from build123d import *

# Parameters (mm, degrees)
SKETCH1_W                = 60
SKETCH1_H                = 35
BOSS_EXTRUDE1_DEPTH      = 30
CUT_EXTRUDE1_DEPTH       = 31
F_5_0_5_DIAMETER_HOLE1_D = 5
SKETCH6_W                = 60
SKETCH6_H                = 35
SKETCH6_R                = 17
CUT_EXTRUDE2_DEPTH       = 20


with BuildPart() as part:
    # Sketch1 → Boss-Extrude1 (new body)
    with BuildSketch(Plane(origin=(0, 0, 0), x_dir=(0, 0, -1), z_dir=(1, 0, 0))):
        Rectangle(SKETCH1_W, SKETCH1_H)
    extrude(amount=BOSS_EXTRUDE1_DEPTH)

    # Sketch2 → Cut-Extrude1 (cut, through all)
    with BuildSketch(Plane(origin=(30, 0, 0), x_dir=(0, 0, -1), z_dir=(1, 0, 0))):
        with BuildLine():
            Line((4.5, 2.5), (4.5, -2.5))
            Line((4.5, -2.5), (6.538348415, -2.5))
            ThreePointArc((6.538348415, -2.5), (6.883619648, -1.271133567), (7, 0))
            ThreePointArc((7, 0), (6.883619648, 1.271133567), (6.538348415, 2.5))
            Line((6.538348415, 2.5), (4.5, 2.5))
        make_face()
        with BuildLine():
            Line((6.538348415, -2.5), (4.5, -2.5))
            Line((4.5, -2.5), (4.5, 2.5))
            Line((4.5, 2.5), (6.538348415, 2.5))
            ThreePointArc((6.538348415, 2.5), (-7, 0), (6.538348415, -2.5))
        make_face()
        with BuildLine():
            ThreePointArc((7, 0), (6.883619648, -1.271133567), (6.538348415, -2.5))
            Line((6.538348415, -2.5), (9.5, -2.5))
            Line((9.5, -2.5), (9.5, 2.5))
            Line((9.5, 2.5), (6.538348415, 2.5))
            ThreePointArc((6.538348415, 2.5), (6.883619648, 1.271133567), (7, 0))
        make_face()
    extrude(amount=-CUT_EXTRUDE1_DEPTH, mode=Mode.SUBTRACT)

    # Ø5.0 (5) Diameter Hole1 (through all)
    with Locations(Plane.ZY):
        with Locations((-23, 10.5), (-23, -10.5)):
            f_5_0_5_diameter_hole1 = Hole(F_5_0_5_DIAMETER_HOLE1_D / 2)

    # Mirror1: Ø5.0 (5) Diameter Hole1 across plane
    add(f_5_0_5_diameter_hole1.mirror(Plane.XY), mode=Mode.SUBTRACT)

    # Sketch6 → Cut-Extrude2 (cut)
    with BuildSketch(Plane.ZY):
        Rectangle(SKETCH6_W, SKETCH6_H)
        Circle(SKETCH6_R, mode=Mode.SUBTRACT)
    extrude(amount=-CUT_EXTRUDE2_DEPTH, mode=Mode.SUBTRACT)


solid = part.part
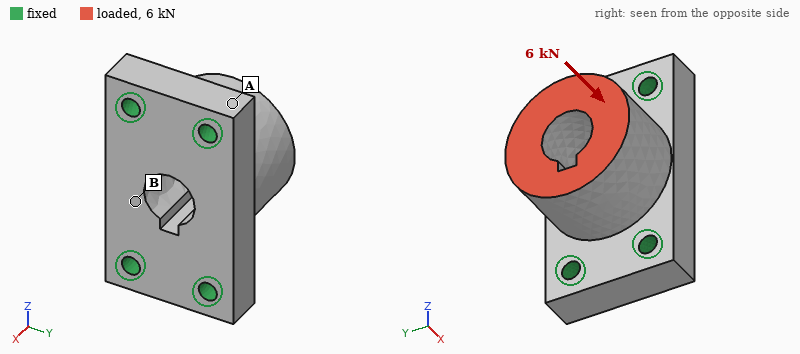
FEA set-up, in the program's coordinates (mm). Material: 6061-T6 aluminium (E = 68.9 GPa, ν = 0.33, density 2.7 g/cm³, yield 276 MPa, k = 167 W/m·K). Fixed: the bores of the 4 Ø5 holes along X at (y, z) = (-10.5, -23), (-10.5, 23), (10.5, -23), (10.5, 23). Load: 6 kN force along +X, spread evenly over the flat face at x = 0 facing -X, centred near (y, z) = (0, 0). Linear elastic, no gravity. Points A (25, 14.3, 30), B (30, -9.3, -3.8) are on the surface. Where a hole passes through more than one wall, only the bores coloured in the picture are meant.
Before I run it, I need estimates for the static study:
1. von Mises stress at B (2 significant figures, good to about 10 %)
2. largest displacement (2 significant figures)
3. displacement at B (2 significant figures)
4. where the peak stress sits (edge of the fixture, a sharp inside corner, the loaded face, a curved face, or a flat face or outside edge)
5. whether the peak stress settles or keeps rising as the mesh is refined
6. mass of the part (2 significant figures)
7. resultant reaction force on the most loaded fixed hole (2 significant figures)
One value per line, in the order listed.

13 MPa
11 µm
8.5 µm
edge of the fixture
keeps rising
90 g
1.6 kN
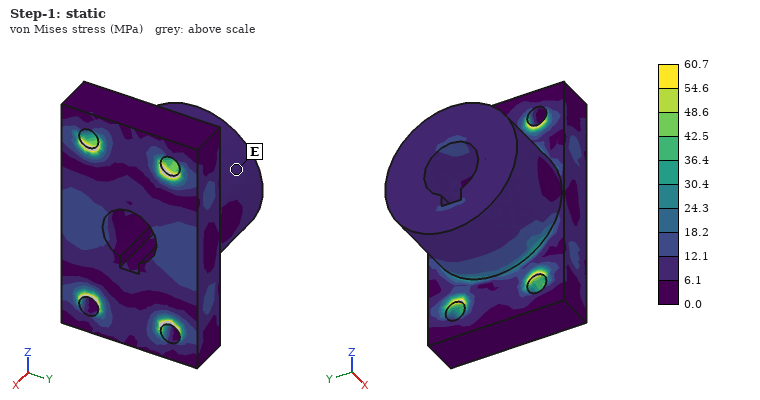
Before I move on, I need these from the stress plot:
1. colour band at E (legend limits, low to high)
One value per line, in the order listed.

6.1 to 12.1 MPa
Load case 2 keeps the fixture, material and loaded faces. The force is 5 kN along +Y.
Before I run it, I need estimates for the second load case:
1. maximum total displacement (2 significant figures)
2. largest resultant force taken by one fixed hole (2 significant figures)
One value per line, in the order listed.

56 µm
3.1 kN
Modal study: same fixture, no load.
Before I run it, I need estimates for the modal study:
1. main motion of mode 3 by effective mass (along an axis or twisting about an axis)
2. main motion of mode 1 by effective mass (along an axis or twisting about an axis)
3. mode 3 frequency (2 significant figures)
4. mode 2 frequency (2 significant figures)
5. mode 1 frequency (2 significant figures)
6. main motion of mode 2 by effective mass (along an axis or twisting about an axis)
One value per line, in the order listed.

along Z
along Y
18 kHz
17 kHz
11 kHz
along X
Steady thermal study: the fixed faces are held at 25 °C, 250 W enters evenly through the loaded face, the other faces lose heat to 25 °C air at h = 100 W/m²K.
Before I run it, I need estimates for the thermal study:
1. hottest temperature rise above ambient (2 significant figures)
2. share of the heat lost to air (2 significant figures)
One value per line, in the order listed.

68 K
8.5 %
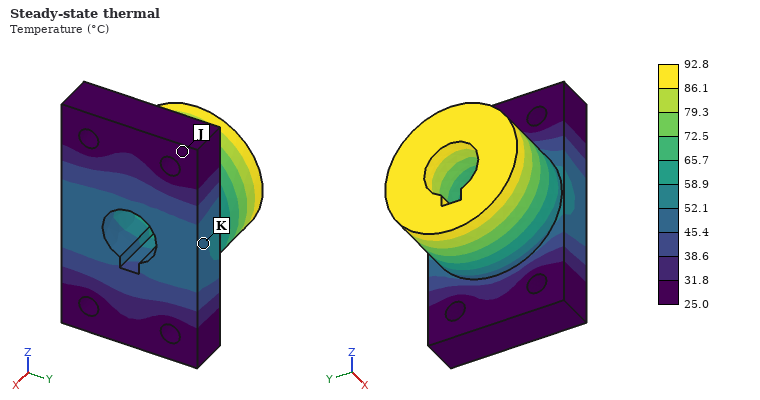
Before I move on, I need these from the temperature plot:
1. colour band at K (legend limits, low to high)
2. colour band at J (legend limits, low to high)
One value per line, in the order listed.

45.4 to 52.1 °C
25.0 to 31.8 °C
